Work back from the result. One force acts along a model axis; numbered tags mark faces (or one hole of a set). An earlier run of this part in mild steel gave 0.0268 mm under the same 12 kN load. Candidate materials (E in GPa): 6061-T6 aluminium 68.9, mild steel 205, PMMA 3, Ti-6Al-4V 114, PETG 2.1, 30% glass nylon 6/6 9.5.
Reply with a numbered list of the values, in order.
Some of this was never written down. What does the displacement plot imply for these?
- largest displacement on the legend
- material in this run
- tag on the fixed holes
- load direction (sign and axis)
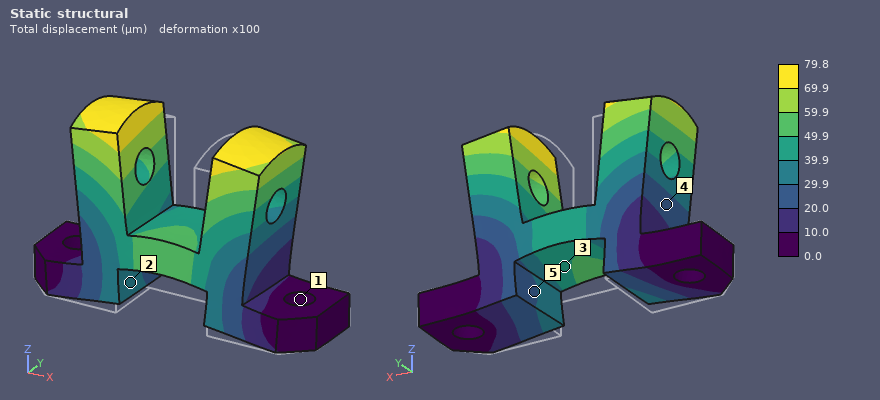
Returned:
1. 79.8 µm
2. 6061-T6 aluminium
3. 1
4. +Z
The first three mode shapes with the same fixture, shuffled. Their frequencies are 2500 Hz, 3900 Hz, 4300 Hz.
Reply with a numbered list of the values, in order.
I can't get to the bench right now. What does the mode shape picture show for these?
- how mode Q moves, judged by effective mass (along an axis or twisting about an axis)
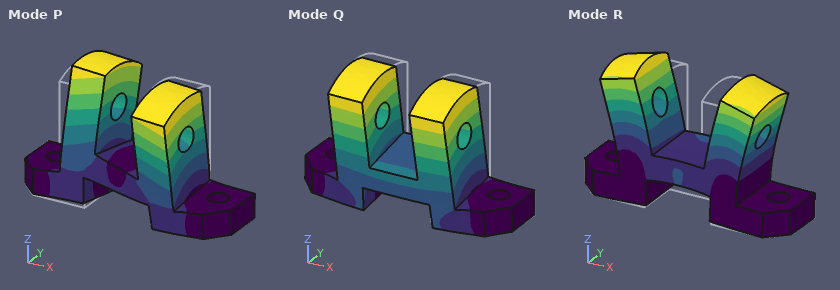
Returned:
1. along Y
